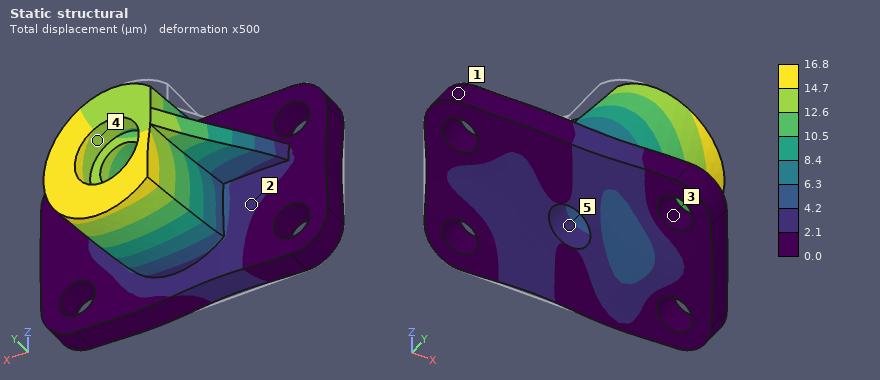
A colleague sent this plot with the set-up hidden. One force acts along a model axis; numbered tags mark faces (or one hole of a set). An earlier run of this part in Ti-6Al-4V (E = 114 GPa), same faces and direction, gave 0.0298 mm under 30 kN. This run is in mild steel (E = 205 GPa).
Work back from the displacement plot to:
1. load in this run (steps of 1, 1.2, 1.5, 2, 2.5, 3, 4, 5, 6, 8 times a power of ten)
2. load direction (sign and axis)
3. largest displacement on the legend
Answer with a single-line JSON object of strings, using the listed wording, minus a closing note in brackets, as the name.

{"load in this run": "30 kN", "load direction": "+X", "largest displacement on the legend": "16.8 µm"}
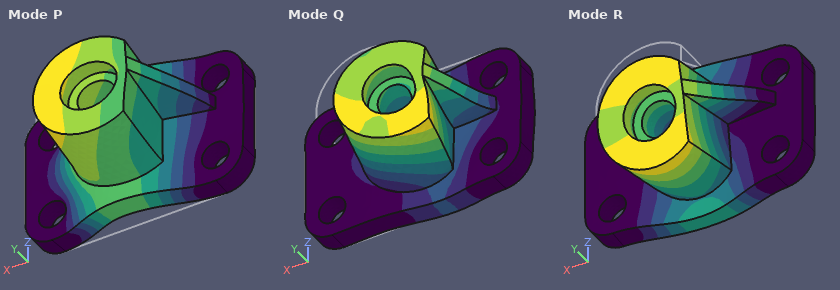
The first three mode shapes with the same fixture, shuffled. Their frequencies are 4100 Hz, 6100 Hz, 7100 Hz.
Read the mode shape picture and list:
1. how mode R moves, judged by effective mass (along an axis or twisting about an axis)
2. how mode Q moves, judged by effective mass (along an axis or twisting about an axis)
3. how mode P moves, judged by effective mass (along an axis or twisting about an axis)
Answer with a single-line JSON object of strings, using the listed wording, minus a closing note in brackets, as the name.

{"how mode R moves, judged by effective mass": "along Z", "how mode Q moves, judged by effective mass": "along X", "how mode P moves, judged by effective mass": "along Y"}
